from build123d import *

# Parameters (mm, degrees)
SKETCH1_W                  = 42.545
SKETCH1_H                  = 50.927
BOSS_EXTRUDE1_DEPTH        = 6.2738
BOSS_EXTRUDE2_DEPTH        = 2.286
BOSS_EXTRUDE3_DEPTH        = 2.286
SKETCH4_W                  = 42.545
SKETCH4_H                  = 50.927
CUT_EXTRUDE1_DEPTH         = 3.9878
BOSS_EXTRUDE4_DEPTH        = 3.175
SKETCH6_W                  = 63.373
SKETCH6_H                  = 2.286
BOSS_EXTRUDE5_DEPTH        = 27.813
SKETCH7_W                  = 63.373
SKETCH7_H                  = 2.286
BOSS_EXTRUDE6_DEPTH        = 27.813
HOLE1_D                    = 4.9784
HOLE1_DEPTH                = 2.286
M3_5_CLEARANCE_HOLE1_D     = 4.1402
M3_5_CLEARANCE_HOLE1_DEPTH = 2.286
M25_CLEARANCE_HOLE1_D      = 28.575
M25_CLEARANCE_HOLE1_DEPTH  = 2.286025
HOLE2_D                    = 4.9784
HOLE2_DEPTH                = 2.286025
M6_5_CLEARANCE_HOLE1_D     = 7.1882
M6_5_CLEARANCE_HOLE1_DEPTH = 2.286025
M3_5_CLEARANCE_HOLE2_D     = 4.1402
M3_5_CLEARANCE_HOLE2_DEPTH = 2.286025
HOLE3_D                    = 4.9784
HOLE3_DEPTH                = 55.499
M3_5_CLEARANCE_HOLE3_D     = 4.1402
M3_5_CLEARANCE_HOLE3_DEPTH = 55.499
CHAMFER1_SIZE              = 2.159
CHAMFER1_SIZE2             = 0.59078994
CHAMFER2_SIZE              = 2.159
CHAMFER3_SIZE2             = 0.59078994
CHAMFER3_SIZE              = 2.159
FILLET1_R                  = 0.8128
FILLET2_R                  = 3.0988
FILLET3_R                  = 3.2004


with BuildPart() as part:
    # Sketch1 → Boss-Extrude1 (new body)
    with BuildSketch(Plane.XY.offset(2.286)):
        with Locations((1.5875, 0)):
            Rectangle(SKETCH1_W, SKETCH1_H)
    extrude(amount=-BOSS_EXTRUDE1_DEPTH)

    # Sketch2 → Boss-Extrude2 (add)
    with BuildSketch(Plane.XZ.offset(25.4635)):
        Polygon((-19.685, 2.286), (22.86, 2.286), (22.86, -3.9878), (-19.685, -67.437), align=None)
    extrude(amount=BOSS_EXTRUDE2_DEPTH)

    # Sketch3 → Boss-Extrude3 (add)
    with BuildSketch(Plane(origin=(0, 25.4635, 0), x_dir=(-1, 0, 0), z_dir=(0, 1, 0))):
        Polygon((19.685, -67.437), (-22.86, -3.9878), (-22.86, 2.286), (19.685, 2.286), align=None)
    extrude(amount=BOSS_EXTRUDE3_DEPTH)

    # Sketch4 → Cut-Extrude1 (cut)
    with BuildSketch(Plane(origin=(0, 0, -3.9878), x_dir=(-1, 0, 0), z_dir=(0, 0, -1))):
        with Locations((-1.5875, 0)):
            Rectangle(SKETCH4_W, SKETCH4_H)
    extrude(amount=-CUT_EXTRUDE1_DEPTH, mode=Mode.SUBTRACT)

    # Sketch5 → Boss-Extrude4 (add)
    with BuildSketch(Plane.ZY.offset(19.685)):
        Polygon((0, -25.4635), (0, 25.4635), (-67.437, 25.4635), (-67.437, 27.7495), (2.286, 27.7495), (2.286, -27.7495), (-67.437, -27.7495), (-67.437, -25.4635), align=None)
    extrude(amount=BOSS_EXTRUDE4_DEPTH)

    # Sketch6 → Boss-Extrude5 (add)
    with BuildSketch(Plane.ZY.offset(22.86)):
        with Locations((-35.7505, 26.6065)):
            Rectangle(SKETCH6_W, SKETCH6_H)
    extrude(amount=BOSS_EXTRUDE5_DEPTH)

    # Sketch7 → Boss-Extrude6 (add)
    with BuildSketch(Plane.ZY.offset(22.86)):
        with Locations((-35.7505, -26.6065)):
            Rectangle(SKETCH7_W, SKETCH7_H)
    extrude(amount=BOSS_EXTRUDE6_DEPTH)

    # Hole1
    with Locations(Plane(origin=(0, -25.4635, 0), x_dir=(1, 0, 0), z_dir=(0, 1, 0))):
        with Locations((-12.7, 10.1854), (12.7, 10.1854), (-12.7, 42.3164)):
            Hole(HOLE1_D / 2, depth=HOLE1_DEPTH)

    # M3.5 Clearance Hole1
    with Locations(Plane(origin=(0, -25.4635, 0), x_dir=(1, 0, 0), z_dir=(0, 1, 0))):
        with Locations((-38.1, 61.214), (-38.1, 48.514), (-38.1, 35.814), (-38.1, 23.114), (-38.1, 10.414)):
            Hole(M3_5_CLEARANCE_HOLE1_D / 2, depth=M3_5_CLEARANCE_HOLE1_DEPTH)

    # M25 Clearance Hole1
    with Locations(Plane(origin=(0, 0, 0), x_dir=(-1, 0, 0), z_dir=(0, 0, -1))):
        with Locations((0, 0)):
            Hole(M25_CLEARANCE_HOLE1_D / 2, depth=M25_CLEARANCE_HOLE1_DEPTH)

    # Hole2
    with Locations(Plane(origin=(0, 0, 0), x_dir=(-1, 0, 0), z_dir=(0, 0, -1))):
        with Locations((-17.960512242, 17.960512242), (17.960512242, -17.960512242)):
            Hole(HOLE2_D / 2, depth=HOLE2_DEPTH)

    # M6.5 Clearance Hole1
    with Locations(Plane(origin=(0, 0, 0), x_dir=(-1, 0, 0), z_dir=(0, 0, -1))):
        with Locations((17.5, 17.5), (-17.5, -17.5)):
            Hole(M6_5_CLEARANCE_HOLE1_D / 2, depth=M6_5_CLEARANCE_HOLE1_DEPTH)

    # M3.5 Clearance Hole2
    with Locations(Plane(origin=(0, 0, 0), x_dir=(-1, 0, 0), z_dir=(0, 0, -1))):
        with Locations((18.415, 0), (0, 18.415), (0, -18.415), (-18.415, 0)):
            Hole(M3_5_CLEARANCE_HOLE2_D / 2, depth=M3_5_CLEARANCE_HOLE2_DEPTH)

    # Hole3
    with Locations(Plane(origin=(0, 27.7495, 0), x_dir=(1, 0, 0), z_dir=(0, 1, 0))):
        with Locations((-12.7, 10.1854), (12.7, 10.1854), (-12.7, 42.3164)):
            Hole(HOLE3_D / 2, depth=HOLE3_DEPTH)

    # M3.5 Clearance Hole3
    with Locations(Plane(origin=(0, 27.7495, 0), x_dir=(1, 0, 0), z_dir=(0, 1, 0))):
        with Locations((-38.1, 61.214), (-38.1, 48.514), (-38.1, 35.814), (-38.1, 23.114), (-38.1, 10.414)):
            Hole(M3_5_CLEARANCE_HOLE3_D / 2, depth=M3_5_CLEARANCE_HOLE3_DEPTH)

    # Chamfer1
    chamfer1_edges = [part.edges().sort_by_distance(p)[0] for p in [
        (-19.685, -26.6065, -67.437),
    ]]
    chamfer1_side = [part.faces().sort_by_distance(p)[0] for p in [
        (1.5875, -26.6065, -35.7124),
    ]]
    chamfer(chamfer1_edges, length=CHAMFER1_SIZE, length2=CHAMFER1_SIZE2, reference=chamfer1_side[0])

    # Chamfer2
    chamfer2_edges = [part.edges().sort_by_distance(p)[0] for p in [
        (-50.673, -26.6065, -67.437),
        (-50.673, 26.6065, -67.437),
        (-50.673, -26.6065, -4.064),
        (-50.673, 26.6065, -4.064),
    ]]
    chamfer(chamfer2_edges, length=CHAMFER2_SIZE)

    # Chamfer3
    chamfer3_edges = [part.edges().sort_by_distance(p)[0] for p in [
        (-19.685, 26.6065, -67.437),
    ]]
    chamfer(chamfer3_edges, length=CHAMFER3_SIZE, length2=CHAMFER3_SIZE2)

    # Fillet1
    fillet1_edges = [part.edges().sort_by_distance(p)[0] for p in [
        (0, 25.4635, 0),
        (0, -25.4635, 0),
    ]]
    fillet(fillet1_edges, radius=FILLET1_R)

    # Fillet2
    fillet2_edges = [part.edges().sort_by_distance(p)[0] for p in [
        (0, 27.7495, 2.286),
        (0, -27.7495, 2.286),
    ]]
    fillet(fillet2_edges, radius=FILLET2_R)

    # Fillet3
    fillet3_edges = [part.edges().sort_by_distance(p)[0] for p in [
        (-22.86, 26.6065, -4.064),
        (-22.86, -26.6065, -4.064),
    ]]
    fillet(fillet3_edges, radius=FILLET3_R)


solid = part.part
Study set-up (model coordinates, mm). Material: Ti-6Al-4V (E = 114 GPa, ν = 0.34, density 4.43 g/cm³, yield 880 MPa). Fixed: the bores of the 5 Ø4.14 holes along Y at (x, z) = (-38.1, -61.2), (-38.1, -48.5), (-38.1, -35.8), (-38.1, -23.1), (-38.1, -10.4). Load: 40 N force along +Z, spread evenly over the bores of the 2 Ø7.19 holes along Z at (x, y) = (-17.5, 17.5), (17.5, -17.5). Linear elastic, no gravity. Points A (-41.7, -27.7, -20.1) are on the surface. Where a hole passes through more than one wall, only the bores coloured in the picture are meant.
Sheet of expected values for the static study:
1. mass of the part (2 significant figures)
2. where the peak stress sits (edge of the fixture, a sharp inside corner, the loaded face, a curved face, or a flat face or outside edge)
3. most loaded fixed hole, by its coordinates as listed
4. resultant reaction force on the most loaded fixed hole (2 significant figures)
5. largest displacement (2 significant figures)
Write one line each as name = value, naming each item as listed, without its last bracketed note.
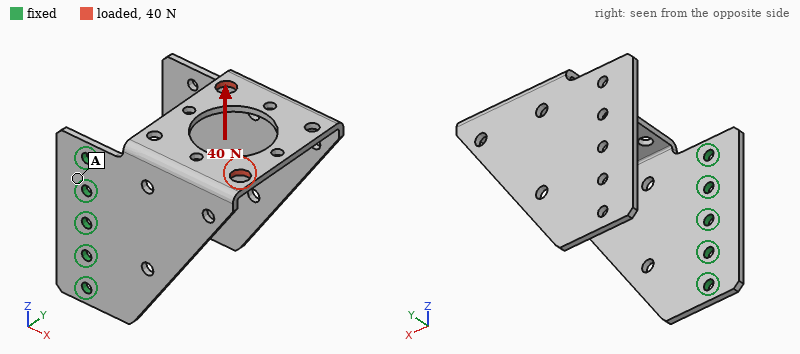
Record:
mass of the part = 85 g
where the peak stress sits = a curved face
most loaded fixed hole, by its coordinates as listed = (-38.1, -10.4)
resultant reaction force on the most loaded fixed hole = 51 N
largest displacement = 1.2 mm
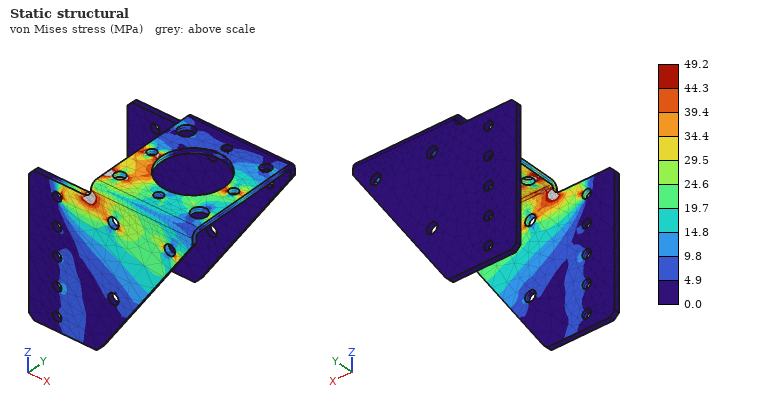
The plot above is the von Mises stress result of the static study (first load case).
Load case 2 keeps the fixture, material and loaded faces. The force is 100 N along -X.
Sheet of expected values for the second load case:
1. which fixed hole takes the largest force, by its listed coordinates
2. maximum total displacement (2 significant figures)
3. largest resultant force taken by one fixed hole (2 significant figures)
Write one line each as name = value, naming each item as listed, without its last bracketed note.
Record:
which fixed hole takes the largest force, by its listed coordinates = (-38.1, -10.4)
maximum total displacement = 1.3 mm
largest resultant force taken by one fixed hole = 98 N
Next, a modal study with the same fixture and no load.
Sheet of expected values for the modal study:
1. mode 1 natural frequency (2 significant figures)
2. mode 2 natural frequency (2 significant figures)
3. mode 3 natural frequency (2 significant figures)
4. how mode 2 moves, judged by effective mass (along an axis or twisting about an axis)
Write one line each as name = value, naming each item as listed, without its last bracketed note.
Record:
mode 1 natural frequency = 100 Hz
mode 2 natural frequency = 140 Hz
mode 3 natural frequency = 260 Hz
how mode 2 moves, judged by effective mass = along X
